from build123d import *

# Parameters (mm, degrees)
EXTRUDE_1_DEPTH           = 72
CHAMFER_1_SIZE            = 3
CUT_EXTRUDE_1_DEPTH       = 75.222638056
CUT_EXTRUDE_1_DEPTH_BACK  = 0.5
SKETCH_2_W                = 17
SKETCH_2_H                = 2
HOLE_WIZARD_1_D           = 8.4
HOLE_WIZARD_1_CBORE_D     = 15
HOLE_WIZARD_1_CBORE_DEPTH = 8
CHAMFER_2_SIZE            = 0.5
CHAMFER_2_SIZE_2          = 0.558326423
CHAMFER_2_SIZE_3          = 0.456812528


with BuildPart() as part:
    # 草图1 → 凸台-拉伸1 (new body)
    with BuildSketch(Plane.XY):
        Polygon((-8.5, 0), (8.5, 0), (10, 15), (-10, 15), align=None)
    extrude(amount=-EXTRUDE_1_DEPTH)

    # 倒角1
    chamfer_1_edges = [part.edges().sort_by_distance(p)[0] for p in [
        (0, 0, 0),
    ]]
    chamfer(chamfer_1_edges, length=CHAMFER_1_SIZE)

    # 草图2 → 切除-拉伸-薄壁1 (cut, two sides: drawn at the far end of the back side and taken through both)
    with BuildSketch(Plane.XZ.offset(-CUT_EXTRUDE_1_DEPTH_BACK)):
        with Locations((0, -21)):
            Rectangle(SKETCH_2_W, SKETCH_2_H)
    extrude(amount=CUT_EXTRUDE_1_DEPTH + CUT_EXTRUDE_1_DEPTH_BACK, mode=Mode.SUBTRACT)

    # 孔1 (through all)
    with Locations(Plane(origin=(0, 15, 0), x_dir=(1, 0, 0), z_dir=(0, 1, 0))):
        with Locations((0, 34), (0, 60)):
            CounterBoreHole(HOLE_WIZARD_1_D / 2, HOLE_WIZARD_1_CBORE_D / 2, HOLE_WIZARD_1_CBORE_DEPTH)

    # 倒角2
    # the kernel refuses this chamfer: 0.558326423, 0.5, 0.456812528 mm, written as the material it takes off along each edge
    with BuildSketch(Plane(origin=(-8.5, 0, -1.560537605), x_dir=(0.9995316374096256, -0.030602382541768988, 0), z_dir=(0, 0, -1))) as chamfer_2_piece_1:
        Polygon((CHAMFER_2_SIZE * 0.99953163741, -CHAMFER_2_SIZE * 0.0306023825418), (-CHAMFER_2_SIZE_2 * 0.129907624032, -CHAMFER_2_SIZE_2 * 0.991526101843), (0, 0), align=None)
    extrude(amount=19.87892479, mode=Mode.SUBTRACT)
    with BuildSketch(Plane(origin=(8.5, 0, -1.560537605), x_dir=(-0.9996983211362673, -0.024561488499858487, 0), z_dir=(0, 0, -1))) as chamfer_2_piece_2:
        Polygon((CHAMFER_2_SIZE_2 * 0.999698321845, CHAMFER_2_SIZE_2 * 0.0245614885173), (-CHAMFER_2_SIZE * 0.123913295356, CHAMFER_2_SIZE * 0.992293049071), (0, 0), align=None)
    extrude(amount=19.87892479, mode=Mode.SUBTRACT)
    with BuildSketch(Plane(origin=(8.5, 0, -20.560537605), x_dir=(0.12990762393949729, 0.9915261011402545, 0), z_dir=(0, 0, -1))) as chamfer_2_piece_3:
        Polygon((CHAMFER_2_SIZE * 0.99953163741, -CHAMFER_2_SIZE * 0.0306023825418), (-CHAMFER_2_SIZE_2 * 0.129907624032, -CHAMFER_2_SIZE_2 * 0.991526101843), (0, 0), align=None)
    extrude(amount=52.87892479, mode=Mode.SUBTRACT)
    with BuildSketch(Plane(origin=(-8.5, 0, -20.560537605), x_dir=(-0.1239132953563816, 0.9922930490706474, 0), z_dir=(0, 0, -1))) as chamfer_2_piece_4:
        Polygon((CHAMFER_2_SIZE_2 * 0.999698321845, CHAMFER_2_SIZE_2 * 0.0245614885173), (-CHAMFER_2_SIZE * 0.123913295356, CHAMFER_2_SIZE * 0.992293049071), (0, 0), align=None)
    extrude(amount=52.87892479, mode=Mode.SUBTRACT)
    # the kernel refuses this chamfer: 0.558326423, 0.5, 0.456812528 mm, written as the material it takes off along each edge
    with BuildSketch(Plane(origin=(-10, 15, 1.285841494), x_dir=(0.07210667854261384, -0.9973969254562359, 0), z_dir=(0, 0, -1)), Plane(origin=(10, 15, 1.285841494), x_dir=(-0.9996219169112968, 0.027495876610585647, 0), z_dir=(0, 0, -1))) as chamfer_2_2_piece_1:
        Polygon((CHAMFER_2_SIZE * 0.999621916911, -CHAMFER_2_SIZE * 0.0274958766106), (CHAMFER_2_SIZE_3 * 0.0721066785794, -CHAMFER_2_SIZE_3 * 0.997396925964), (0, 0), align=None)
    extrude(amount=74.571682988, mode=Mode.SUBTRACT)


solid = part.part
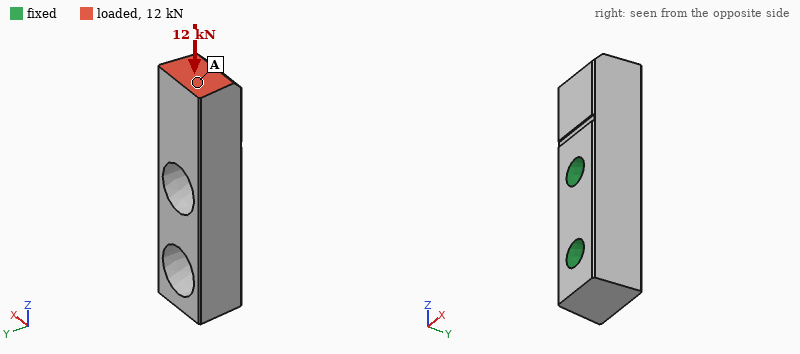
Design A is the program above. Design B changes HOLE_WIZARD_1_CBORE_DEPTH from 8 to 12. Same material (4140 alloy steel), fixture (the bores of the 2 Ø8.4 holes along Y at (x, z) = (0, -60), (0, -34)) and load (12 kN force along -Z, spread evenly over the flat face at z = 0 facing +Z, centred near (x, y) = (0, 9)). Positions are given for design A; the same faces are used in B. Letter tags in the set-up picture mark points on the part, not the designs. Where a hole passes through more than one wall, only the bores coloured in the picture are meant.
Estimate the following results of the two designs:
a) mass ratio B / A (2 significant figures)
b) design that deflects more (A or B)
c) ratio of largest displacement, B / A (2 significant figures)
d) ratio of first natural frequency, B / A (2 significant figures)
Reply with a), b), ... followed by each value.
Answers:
a) 0.94
b) B
c) 1.7
d) 0.81
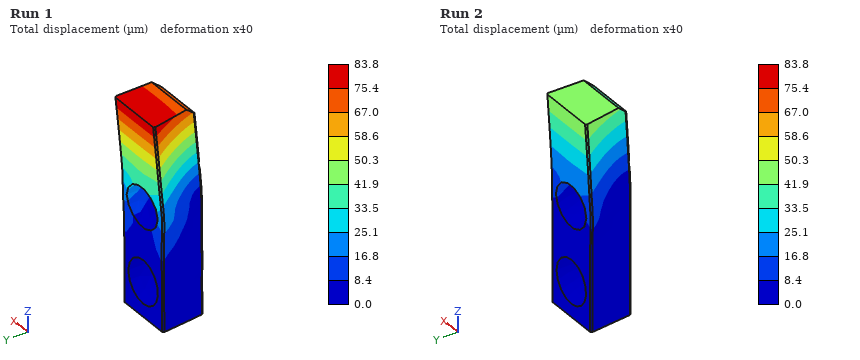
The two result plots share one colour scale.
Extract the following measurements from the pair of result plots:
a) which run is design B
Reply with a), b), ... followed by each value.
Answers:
a) Run 1
